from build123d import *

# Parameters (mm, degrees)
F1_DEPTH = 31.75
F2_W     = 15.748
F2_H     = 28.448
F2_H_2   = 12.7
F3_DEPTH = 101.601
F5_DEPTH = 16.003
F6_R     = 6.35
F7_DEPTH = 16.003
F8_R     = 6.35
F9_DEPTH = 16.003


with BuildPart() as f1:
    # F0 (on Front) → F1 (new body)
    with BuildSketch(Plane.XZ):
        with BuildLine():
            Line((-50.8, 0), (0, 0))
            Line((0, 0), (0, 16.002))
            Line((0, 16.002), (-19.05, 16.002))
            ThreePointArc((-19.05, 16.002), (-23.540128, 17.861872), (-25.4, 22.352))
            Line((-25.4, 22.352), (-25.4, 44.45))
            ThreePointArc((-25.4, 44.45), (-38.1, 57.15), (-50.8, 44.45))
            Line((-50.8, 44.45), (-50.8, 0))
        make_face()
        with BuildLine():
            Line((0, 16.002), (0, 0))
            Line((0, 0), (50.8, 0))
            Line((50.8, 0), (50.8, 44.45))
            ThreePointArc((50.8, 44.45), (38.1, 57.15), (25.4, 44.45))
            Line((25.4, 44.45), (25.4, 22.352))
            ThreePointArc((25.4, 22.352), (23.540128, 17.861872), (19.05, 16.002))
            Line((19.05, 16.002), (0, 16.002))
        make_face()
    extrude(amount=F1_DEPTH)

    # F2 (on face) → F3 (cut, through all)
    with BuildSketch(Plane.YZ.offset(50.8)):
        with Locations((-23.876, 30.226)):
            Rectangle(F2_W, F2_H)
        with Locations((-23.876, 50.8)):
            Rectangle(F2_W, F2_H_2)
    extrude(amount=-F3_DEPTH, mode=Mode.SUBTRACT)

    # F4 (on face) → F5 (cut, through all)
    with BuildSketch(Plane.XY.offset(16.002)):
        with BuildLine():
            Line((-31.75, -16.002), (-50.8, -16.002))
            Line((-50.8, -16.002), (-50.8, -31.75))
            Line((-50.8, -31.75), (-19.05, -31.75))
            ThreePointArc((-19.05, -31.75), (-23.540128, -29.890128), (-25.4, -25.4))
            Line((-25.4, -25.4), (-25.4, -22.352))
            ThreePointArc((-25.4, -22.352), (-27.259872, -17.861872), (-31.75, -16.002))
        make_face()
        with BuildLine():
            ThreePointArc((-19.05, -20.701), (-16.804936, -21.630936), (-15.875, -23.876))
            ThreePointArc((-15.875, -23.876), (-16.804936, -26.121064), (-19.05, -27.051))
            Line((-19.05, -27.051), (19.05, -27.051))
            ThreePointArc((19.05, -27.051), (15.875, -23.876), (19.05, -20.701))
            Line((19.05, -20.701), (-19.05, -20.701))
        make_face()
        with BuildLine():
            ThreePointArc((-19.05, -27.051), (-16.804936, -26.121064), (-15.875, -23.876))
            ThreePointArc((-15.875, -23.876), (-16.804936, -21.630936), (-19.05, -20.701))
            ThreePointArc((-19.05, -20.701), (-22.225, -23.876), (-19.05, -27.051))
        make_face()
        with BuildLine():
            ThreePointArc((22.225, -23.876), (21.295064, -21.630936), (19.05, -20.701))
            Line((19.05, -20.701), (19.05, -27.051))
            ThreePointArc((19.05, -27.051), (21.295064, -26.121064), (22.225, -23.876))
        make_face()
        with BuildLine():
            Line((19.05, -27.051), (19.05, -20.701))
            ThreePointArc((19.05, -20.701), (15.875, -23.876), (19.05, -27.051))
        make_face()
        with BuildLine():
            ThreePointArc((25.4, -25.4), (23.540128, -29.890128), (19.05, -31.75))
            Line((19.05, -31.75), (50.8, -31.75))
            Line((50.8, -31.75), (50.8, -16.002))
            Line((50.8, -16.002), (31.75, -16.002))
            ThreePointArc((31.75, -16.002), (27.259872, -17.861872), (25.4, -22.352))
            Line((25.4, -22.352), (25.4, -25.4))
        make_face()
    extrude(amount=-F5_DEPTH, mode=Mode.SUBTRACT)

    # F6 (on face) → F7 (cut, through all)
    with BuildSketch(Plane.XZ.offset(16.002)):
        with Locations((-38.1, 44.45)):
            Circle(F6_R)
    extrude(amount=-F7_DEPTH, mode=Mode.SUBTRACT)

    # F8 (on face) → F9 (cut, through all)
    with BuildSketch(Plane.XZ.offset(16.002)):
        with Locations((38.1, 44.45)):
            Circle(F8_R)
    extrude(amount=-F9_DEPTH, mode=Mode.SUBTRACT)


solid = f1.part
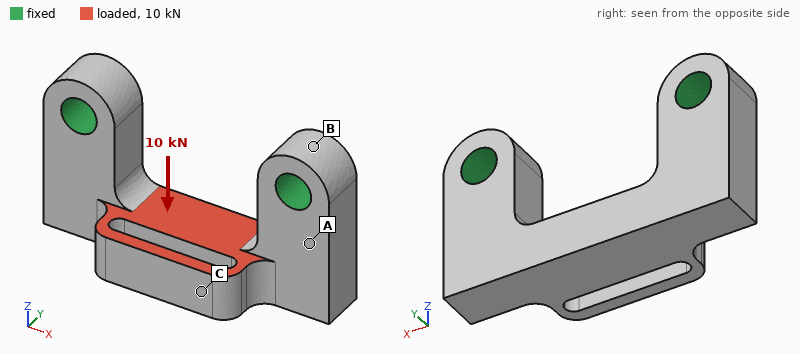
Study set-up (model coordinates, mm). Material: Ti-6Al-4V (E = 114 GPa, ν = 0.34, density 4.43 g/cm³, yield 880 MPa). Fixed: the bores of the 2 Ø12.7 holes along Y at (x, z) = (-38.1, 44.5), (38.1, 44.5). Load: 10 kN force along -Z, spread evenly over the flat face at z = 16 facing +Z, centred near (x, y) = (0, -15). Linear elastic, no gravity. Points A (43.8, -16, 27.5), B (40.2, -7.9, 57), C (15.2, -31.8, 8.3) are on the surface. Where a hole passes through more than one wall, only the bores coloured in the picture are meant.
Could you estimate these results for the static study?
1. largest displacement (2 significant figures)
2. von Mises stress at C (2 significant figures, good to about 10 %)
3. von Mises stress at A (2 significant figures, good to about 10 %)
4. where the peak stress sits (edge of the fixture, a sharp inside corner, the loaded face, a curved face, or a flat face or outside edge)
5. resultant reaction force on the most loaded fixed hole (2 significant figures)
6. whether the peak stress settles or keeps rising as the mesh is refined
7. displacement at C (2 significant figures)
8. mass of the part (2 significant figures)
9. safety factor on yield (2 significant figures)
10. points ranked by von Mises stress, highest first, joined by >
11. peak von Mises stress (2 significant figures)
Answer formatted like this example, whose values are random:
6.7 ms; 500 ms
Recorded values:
83 µm; 25 MPa; 34 MPa; a curved face; 5.7 kN; settles; 68 µm; 270 g; 5.1; A > C > B; 170 MPa
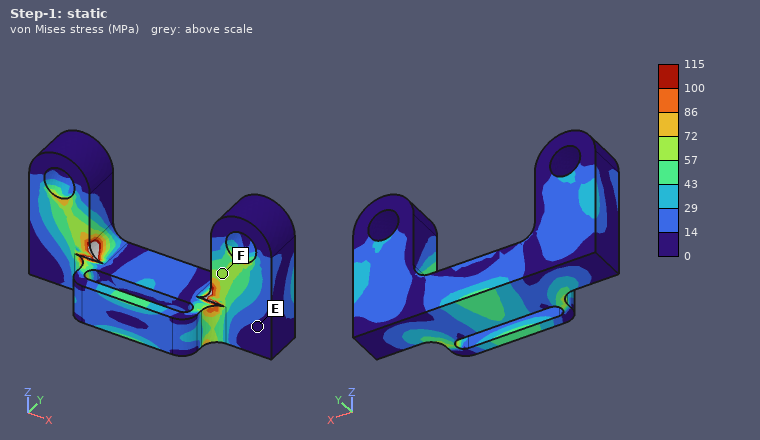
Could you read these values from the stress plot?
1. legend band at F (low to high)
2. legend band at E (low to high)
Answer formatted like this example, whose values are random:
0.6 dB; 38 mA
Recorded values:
57 to 72 MPa; 0 to 14 MPa
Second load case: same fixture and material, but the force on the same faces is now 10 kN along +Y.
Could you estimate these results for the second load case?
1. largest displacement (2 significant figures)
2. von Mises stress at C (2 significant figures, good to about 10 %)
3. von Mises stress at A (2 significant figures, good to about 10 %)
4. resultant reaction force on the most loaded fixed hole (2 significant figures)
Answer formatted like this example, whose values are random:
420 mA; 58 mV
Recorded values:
0.13 mm; 80 MPa; 54 MPa; 5.0 kN
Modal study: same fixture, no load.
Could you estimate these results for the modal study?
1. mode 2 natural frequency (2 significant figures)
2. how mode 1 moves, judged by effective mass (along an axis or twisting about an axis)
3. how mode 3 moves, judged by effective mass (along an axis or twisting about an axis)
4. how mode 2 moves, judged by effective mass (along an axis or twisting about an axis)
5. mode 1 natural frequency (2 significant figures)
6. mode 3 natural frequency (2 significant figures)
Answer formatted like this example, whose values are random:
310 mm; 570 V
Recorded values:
7000 Hz; along Y; along X; along X; 4100 Hz; 7800 Hz
